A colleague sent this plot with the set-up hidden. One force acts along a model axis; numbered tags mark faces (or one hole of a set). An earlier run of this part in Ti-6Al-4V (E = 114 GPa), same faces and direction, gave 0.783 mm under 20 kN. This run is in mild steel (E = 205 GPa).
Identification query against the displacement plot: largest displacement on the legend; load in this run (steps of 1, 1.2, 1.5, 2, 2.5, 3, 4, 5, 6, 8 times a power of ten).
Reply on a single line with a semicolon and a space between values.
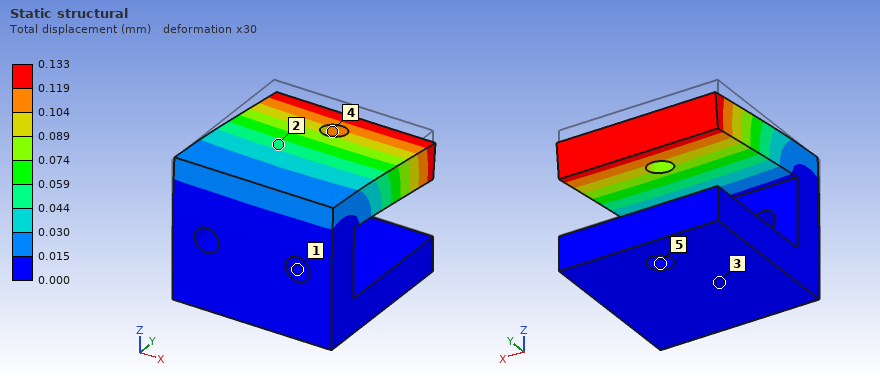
0.133 mm; 6 kN
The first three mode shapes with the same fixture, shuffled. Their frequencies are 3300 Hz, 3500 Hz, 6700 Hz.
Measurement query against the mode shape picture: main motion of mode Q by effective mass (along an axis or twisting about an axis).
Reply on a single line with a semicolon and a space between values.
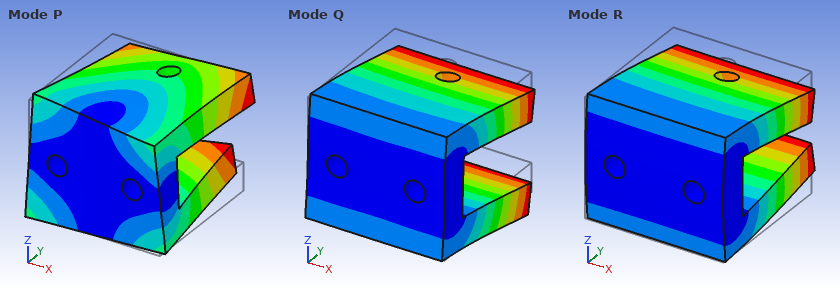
along Z
